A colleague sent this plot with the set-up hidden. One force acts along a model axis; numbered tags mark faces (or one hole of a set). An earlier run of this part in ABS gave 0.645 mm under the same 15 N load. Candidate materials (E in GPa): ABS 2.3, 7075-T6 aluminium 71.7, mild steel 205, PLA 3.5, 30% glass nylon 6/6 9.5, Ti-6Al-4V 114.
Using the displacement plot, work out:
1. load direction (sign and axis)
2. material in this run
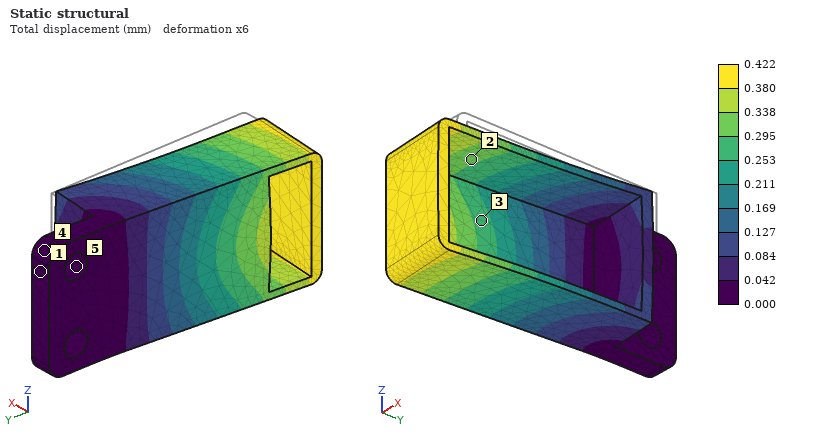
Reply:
-X
PLA
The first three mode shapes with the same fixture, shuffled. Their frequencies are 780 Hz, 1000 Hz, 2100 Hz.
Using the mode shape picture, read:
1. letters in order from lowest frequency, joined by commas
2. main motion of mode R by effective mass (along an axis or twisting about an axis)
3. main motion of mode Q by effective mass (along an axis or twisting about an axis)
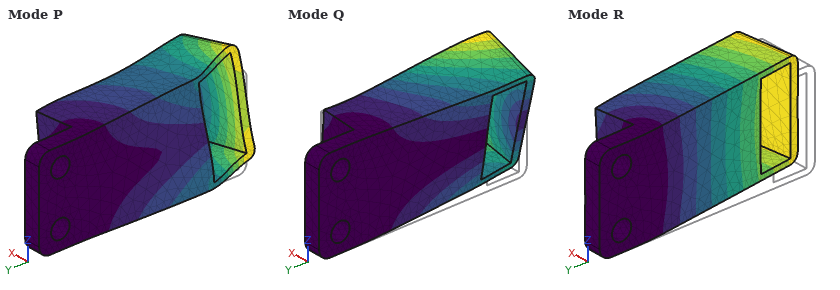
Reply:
R, Q, P
along X
along Z
